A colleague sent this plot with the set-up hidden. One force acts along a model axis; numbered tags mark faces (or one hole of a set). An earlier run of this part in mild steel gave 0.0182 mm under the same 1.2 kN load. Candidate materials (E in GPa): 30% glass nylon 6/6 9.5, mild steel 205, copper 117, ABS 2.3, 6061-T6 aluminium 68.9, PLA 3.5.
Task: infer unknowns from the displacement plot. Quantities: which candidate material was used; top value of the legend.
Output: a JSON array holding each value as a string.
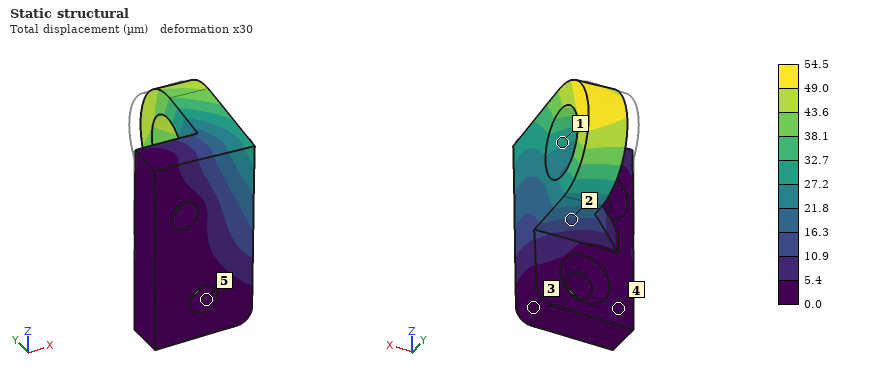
["6061-T6 aluminium", "54.5 µm"]
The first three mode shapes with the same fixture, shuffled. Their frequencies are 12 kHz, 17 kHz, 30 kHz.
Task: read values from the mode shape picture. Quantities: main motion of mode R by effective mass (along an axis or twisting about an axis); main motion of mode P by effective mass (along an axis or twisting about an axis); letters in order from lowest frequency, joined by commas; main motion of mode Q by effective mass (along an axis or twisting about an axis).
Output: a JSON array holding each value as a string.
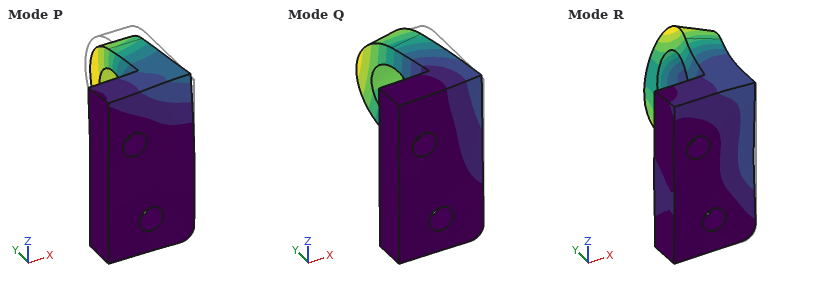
["along Y", "along Z", "Q, P, R", "along X"]
